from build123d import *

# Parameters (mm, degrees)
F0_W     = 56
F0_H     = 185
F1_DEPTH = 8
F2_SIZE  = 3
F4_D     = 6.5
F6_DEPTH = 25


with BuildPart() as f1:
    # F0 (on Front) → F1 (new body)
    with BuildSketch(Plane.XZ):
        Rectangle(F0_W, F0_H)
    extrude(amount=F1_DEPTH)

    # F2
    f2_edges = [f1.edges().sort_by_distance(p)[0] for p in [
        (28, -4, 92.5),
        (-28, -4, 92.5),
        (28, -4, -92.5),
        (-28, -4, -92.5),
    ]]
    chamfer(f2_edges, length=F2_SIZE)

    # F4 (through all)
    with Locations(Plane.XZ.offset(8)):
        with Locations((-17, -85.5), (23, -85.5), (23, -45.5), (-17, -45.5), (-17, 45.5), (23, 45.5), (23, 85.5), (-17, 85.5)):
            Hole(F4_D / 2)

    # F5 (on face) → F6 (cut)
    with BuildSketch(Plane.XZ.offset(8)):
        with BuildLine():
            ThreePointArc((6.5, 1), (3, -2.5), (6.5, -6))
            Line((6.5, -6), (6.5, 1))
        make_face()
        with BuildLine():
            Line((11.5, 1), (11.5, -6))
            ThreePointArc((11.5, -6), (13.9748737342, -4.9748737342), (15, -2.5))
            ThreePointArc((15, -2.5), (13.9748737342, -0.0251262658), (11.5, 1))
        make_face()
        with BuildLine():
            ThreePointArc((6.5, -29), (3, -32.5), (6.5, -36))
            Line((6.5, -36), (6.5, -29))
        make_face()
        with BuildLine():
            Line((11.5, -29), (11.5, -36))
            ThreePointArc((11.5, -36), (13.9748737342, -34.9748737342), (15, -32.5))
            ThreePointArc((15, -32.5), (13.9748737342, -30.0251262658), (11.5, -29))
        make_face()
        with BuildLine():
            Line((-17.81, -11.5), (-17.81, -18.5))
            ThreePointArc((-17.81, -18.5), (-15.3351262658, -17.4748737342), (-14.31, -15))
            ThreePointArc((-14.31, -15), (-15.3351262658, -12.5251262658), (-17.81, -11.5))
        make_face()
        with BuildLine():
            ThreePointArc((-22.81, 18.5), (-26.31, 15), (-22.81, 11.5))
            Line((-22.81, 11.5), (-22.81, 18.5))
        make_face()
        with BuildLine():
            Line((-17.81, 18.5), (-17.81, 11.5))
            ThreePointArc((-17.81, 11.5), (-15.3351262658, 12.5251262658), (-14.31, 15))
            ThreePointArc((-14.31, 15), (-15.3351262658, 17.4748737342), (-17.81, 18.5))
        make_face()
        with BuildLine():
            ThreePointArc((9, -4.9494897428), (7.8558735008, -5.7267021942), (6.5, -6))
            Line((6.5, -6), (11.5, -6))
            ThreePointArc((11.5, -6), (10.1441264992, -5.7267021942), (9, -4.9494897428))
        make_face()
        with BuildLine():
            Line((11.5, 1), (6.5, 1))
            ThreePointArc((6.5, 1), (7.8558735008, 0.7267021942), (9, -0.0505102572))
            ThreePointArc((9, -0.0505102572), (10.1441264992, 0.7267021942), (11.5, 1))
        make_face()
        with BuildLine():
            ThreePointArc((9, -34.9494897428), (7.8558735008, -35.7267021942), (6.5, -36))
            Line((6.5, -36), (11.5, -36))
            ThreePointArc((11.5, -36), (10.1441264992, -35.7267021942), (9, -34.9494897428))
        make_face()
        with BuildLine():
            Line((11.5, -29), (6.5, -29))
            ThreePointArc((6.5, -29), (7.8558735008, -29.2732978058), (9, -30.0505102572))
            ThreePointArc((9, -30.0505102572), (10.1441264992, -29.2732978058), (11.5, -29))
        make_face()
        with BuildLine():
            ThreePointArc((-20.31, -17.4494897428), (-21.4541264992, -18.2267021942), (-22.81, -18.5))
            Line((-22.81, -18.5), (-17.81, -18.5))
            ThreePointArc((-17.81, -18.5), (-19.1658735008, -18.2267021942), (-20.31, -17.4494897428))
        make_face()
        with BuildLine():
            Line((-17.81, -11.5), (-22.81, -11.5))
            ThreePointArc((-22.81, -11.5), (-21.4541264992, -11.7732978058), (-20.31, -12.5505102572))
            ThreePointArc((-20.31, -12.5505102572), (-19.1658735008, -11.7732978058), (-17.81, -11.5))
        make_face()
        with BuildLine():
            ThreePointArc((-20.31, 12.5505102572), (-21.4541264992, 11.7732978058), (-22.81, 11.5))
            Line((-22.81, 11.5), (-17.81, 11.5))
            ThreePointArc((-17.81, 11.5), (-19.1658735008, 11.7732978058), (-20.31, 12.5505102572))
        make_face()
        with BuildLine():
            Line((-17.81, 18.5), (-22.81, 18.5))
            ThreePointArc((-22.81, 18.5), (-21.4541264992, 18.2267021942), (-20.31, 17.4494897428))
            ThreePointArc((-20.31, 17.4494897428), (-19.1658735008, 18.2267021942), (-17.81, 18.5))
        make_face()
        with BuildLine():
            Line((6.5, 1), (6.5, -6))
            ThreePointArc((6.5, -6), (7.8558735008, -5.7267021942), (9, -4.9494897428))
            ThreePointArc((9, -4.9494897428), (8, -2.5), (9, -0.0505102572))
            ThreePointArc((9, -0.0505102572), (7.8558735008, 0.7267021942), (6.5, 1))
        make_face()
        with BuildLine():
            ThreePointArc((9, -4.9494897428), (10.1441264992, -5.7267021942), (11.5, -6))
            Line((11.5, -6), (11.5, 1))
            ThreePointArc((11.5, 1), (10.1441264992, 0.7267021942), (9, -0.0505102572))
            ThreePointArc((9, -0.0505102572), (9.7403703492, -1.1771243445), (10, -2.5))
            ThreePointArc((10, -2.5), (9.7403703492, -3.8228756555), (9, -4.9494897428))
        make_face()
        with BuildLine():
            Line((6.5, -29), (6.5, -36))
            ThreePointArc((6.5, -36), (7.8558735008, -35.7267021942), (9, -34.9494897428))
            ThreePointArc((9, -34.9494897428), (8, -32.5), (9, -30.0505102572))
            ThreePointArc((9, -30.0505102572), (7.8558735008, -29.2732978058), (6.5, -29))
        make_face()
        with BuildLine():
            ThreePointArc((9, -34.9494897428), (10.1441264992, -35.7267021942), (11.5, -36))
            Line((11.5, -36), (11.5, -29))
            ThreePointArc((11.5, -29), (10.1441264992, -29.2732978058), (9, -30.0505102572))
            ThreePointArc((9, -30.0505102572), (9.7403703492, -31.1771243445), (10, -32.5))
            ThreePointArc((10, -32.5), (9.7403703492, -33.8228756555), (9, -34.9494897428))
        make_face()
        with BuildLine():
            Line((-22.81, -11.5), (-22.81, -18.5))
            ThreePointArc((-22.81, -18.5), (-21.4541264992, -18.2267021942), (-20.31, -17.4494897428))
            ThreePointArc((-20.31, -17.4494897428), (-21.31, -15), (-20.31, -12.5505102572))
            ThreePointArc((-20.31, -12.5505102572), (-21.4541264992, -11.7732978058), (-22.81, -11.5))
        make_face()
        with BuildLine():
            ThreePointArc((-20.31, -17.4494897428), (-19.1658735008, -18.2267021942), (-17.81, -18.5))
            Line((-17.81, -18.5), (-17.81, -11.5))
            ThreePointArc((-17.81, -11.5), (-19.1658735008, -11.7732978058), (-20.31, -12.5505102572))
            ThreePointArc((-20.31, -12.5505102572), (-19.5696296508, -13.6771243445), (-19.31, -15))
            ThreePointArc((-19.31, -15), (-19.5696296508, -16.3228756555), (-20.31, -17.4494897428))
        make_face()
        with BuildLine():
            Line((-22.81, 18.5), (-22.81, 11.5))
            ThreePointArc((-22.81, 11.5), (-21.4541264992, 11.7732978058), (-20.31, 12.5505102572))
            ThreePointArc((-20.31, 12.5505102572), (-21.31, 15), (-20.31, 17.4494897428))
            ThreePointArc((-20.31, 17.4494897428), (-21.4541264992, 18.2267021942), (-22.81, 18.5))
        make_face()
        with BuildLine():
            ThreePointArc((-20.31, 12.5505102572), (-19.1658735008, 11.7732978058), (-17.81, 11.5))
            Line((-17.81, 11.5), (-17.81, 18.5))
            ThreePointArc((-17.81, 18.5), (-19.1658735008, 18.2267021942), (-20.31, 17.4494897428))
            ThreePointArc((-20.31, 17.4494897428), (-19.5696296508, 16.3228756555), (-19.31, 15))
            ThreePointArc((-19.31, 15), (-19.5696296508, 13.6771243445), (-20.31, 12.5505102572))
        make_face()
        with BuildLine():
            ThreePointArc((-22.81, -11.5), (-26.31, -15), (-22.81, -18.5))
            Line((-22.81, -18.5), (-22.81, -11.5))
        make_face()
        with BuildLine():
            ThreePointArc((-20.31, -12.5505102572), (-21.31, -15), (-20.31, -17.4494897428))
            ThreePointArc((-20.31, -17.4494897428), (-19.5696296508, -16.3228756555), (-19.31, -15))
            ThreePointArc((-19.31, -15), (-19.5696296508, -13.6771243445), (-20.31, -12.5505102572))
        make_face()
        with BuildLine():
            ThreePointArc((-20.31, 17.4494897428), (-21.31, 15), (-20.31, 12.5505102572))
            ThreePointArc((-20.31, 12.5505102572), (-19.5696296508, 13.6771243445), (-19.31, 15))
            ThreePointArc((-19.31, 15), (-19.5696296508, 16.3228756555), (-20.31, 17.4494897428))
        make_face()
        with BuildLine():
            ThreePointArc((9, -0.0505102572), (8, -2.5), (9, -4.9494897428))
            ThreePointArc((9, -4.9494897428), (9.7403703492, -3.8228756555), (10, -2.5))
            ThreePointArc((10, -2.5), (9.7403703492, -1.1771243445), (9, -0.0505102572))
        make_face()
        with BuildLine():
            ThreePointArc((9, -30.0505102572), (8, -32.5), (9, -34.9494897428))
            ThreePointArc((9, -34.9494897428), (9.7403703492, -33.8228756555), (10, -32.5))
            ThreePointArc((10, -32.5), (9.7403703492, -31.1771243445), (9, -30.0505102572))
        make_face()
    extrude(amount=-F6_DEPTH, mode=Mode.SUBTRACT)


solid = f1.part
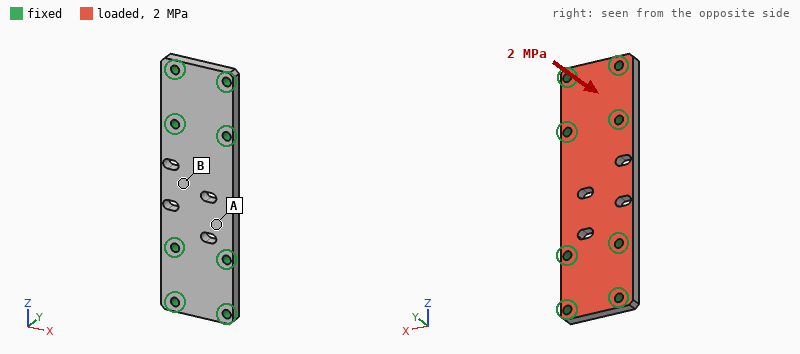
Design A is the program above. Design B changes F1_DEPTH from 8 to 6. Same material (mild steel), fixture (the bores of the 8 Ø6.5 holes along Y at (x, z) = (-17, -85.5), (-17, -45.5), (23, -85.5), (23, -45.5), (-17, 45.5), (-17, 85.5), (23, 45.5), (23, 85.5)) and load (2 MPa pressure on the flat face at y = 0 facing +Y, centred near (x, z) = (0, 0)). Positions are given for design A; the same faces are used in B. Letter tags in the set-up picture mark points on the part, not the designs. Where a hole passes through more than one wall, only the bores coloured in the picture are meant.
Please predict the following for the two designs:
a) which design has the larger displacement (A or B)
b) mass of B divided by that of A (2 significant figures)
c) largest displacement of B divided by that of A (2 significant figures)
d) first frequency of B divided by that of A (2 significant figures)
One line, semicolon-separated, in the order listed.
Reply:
B; 0.75; 2.2; 0.78
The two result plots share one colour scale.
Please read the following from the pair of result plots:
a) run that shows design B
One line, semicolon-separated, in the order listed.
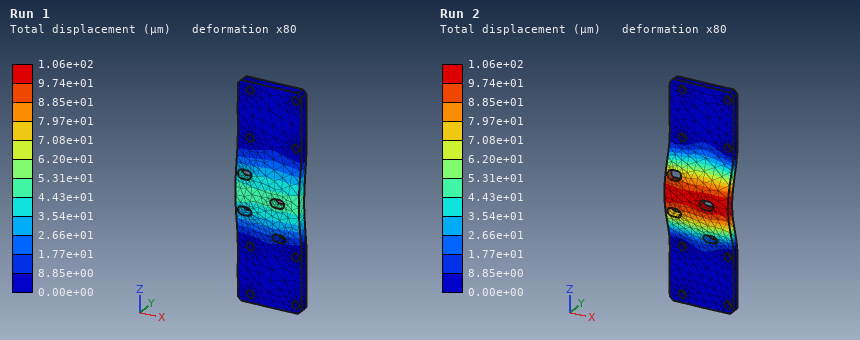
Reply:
Run 2
